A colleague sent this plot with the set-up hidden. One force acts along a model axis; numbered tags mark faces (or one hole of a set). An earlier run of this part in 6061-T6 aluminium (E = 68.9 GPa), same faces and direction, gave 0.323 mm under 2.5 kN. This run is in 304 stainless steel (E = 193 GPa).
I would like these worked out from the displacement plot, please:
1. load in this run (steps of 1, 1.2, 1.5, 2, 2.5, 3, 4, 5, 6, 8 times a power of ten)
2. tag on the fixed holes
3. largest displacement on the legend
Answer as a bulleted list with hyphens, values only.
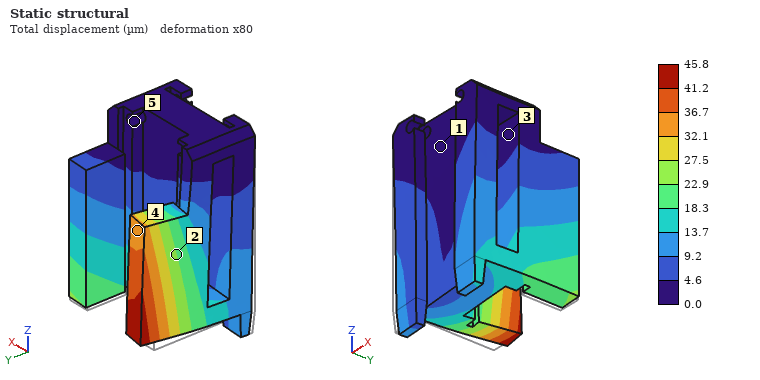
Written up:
- 1 kN
- 5
- 45.8 µm
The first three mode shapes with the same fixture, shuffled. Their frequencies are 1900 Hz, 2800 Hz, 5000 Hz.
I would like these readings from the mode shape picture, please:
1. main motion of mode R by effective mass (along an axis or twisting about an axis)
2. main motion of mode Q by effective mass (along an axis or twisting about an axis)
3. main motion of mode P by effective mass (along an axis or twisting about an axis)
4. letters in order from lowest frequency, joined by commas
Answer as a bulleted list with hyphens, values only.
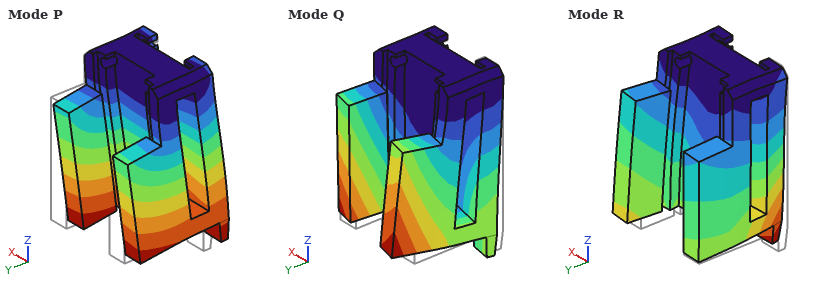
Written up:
- along X
- along X
- along Y
- P, Q, R
